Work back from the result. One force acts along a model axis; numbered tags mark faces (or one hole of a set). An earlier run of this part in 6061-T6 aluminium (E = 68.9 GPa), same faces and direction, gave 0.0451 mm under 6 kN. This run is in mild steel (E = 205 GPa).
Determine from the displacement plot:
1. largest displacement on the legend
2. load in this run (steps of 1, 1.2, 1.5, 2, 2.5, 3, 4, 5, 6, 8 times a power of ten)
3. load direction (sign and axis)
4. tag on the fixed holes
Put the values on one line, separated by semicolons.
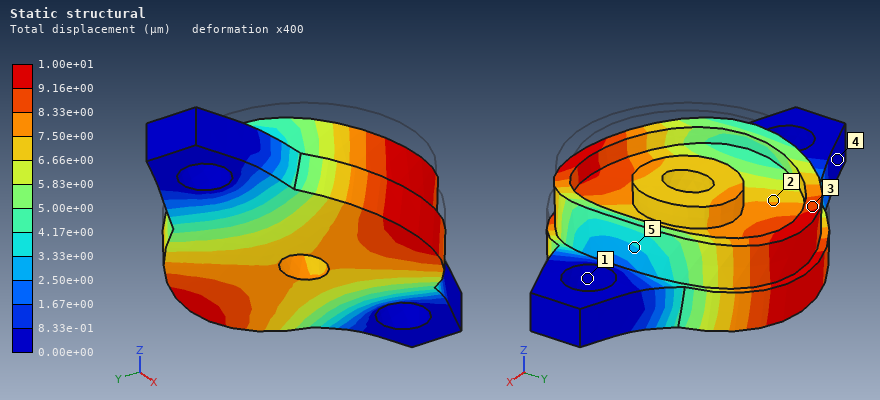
1.00e+01 µm; 4 kN; -Z; 1
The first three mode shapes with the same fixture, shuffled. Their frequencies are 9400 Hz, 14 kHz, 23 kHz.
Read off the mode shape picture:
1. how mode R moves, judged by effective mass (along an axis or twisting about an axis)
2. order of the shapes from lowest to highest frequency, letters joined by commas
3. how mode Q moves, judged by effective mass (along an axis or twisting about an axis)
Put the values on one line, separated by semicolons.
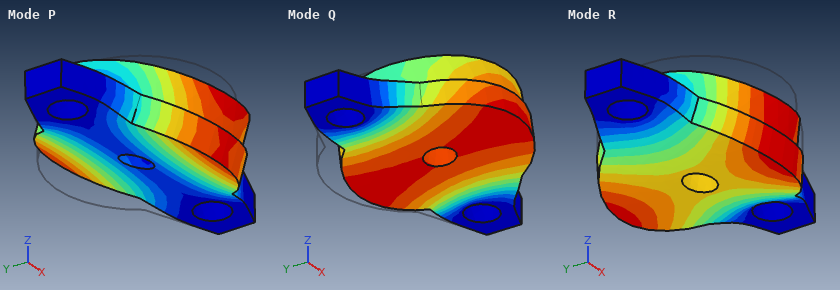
along Z; P, R, Q; along Y
